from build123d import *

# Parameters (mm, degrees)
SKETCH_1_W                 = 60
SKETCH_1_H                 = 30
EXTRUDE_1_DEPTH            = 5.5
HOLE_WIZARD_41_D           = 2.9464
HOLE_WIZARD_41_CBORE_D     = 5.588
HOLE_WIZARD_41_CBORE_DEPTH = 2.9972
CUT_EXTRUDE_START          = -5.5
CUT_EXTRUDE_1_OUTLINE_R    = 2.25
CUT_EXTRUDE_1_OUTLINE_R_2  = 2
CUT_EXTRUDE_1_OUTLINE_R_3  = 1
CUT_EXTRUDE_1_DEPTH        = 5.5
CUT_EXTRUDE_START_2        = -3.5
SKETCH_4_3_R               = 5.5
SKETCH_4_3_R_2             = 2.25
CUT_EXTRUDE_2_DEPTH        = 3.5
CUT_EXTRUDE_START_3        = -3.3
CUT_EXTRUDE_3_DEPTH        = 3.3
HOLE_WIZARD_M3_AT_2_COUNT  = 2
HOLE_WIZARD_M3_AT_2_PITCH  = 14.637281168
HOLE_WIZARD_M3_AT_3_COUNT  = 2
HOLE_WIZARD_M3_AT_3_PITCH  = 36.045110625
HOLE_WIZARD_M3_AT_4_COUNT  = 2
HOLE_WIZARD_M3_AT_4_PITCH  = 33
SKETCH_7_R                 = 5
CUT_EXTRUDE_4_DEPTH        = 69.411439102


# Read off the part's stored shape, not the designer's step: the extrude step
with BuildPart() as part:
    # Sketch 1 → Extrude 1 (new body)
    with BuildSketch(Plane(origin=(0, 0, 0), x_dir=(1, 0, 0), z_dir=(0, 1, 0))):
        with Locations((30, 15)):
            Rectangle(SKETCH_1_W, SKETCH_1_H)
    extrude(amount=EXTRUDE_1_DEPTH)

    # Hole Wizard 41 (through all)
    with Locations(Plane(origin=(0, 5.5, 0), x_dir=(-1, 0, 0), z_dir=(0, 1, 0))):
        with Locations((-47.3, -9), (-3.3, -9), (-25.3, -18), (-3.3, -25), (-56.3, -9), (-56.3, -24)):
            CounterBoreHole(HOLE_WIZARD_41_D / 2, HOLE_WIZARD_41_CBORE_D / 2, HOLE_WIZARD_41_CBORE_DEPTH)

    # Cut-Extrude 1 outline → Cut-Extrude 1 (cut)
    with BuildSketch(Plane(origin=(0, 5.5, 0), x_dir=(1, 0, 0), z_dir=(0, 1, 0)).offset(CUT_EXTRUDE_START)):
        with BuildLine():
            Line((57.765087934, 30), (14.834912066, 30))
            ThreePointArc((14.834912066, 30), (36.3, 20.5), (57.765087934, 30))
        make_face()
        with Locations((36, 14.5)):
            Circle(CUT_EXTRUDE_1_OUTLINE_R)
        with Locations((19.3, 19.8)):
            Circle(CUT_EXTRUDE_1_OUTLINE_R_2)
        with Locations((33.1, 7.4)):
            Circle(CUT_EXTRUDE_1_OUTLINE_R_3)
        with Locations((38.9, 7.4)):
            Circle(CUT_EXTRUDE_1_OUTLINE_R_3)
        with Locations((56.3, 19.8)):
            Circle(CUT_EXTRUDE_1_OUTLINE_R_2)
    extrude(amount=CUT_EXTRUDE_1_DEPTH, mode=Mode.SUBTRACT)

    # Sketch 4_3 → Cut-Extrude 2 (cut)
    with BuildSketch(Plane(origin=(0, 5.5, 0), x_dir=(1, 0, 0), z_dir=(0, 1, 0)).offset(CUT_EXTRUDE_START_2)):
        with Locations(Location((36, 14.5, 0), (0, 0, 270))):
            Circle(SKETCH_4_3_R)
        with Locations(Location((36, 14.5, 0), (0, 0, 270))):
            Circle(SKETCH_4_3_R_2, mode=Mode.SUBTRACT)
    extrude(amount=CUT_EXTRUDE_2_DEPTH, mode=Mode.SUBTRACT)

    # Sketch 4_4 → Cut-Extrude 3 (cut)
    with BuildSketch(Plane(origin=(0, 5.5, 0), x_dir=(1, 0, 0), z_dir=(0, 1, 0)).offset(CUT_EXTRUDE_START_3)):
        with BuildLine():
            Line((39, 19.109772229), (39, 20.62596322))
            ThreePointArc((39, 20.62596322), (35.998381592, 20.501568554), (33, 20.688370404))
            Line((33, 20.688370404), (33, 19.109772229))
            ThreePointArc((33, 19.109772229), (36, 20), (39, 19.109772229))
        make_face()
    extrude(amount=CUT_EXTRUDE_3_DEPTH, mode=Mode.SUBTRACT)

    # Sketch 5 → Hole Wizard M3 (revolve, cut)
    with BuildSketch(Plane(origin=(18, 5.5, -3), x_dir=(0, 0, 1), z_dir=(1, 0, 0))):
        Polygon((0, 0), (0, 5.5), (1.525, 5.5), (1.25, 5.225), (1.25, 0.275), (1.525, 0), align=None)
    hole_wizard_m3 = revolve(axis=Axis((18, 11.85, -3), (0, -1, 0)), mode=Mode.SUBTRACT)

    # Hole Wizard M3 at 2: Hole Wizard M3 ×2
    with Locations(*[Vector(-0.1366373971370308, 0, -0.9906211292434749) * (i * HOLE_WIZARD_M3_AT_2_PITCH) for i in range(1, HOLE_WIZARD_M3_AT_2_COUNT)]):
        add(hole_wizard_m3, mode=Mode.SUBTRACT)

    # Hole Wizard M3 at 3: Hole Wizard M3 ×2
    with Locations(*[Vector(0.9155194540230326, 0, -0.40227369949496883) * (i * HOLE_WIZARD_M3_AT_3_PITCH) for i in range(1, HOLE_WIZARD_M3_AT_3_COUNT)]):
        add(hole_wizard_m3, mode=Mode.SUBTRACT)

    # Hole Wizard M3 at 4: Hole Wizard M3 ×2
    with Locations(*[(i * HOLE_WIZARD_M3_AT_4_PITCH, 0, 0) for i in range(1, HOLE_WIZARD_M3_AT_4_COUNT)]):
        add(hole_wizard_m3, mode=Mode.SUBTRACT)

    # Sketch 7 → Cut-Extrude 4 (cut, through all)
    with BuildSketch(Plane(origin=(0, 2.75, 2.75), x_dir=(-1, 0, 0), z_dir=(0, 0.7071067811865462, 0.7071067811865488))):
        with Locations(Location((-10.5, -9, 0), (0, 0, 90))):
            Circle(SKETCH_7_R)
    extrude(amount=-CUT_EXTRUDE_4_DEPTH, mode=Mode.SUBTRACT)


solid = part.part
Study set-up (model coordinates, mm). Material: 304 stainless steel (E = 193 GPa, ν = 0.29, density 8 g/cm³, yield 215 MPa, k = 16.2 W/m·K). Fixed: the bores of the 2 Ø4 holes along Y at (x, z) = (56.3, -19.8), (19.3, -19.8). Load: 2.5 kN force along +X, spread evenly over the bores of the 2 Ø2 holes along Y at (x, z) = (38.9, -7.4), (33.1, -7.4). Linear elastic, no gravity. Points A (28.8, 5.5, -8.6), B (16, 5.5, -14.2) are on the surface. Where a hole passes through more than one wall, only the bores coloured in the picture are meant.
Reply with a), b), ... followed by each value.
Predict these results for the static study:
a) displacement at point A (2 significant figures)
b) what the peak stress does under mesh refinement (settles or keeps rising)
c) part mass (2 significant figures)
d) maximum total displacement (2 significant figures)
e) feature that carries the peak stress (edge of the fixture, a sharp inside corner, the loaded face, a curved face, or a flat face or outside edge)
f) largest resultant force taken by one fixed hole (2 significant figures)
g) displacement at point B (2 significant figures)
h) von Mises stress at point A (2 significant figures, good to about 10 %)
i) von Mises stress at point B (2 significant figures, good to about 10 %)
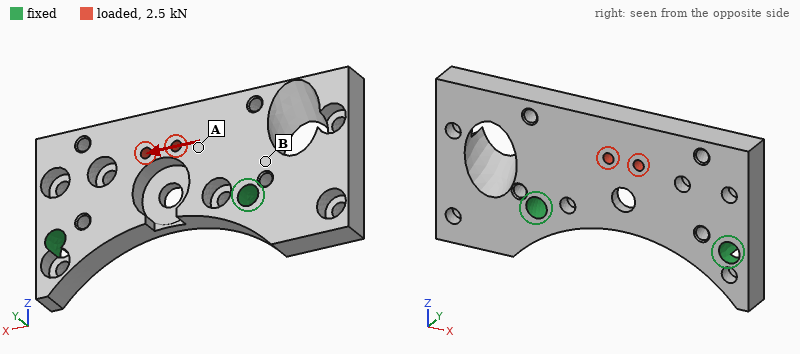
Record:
a) 4.3 µm
b) keeps rising
c) 52 g
d) 6.4 µm
e) edge of the fixture
f) 1.4 kN
g) 1.8 µm
h) 36 MPa
i) 15 MPa
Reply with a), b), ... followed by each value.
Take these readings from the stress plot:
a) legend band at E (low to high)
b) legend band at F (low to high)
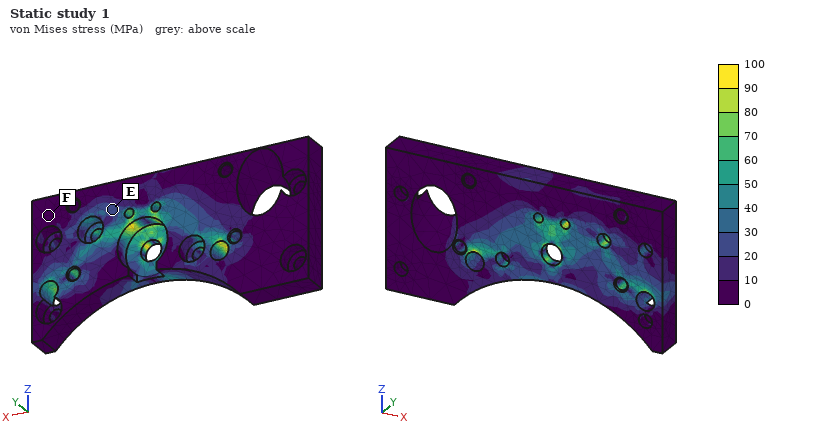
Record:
a) 20 to 30 MPa
b) 0 to 10 MPa
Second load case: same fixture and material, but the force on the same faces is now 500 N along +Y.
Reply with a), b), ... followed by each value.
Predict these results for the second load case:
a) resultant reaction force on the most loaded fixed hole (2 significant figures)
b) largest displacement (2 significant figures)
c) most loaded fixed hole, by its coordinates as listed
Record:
a) 300 N
b) 17 µm
c) (19.3, -19.8)
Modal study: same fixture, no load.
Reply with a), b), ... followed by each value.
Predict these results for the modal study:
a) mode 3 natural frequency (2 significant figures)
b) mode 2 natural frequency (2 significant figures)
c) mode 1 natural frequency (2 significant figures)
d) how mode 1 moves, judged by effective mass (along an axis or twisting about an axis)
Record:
a) 12 kHz
b) 7800 Hz
c) 6900 Hz
d) along Y
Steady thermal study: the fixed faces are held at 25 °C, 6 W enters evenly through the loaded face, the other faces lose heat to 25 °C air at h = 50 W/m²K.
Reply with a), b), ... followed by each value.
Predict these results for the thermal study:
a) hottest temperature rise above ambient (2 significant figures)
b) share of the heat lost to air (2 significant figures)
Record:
a) 46 K
b) 44 %
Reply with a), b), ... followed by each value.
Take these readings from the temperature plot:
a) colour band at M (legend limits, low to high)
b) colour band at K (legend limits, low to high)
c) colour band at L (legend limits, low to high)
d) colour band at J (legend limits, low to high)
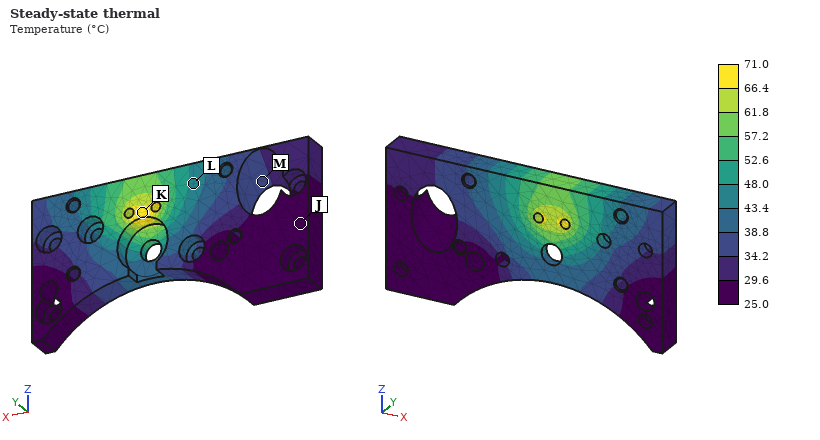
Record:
a) 34.2 to 38.8 °C
b) 66.4 to 71.0 °C
c) 43.4 to 48.0 °C
d) 25.0 to 29.6 °C
